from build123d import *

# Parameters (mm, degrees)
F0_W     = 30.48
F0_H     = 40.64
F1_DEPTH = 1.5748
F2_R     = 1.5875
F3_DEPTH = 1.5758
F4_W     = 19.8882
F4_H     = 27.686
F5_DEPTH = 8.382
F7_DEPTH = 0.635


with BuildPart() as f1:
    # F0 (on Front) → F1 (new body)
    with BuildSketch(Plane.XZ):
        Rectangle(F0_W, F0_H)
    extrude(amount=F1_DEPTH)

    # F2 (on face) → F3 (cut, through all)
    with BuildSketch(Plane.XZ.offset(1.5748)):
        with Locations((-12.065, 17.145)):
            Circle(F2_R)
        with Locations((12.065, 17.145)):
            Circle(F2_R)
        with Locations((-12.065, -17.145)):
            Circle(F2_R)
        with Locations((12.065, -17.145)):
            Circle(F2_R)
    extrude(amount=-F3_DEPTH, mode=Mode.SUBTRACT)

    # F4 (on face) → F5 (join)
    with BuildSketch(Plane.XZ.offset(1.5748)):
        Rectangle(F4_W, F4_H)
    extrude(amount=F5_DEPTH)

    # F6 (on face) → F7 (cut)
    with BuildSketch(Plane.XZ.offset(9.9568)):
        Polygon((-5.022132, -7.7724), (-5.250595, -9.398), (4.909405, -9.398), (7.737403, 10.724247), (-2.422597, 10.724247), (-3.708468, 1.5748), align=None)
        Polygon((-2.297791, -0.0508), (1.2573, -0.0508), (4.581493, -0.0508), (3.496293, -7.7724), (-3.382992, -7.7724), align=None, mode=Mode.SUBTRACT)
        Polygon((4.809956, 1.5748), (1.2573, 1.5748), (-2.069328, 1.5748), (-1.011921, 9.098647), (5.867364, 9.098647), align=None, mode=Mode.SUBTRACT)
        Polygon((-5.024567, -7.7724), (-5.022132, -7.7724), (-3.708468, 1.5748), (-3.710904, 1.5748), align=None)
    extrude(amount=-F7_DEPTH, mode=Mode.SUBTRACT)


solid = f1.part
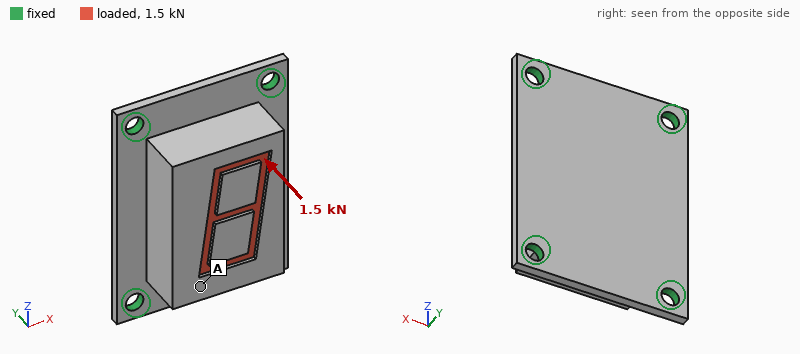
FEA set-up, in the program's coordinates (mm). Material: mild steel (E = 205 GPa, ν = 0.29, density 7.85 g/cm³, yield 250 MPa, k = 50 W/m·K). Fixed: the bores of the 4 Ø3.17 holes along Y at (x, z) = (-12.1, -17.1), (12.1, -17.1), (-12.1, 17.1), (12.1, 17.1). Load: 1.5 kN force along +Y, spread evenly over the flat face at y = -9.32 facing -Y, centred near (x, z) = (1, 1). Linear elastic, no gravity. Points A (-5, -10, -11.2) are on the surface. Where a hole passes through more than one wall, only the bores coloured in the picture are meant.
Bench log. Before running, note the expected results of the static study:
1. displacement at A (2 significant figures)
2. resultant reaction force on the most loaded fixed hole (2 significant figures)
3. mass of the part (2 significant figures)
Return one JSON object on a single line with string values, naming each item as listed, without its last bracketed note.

{"displacement at A": "8.0 µm", "resultant reaction force on the most loaded fixed hole": "510 N", "mass of the part": "51 g"}
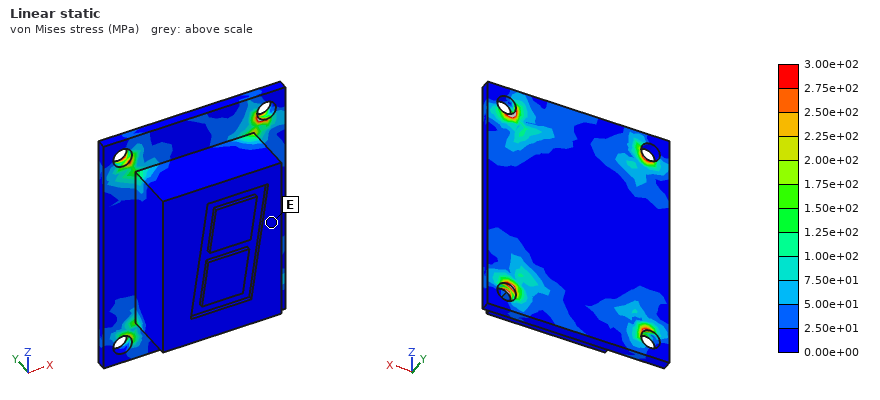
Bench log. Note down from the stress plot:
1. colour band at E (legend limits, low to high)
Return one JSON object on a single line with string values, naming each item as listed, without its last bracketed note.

{"colour band at E": "0.00e+00 to 2.50e+01 MPa"}
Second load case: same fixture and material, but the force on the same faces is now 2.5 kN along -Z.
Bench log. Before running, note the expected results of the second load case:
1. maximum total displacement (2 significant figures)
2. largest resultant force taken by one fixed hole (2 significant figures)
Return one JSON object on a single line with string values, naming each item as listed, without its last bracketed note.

{"maximum total displacement": "10 µm", "largest resultant force taken by one fixed hole": "770 N"}
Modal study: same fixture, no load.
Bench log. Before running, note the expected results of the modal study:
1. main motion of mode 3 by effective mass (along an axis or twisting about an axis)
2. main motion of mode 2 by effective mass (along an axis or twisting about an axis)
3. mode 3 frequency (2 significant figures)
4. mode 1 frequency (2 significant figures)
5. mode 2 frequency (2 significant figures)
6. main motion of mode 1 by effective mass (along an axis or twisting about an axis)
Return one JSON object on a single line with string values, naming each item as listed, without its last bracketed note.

{"main motion of mode 3 by effective mass": "along Z", "main motion of mode 2 by effective mass": "along X", "mode 3 frequency": "15 kHz", "mode 1 frequency": "9500 Hz", "mode 2 frequency": "12 kHz", "main motion of mode 1 by effective mass": "along Y"}
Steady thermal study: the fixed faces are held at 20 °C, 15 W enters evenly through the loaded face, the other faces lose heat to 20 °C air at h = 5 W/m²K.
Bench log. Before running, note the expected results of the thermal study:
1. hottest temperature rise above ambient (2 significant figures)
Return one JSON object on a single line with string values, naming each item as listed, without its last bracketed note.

{"hottest temperature rise above ambient": "38 K"}
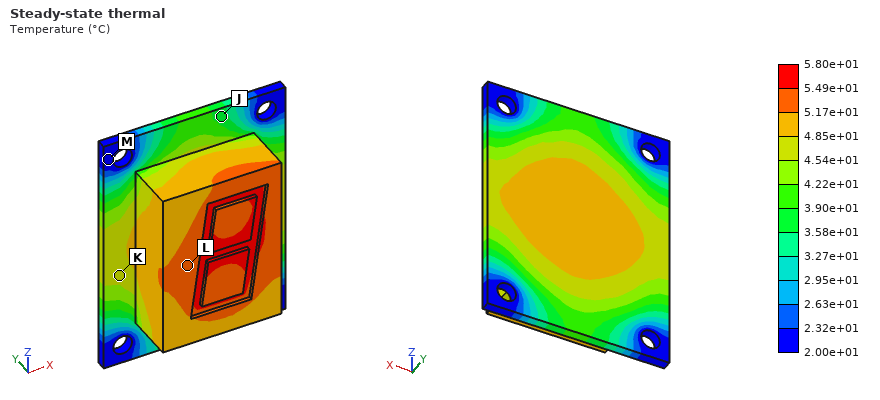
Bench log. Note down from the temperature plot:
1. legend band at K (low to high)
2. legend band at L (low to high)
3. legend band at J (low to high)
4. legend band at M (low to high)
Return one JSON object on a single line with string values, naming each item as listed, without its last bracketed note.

{"legend band at K": "4.54e+01 to 4.85e+01 °C", "legend band at L": "5.17e+01 to 5.49e+01 °C", "legend band at J": "3.58e+01 to 3.90e+01 °C", "legend band at M": "2.00e+01 to 2.32e+01 °C"}
